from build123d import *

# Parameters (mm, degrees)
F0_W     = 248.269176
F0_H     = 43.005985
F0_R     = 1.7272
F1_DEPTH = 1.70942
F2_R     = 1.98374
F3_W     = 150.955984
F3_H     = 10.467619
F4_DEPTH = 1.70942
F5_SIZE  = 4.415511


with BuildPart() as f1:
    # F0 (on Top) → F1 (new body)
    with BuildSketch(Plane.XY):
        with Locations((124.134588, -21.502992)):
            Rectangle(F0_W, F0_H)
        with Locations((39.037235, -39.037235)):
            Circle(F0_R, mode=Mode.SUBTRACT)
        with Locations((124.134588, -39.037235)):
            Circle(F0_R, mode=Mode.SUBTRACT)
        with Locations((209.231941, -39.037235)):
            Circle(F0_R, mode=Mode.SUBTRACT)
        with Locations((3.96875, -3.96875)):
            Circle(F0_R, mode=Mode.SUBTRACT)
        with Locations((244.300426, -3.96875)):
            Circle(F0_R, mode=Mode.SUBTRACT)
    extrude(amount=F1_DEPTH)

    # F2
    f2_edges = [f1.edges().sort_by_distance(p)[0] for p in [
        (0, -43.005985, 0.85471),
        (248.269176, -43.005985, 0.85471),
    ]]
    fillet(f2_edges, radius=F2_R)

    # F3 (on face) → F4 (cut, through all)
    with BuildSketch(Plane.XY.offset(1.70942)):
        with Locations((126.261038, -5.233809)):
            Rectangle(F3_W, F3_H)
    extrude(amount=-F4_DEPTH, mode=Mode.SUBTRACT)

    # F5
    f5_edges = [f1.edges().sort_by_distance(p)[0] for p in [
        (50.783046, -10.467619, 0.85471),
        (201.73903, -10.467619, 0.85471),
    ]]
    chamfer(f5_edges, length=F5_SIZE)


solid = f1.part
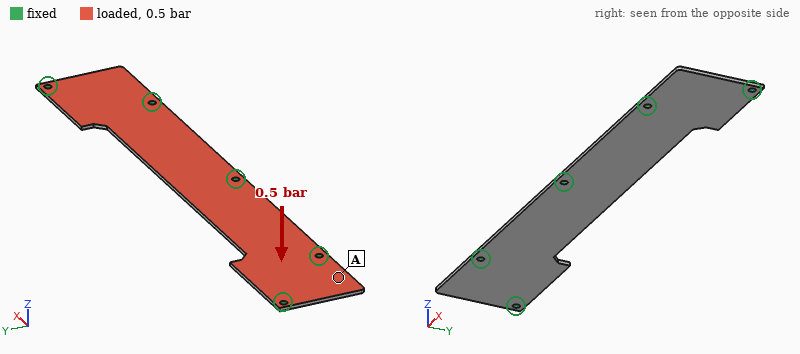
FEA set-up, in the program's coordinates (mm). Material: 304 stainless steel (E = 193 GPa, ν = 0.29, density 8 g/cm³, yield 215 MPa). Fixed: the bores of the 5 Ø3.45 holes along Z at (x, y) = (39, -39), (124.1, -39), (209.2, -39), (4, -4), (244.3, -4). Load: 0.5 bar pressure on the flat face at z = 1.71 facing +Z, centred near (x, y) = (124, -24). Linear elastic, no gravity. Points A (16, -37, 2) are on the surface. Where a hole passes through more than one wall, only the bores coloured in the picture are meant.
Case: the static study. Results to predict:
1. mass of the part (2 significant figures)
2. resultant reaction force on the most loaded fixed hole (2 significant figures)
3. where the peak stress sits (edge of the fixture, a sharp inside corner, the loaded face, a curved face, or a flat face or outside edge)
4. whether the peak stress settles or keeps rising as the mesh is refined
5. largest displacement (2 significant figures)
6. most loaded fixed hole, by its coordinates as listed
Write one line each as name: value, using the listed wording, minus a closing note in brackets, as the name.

mass of the part: 120 g
resultant reaction force on the most loaded fixed hole: 140 N
where the peak stress sits: edge of the fixture
whether the peak stress settles or keeps rising as the mesh is refined: keeps rising
largest displacement: 0.21 mm
most loaded fixed hole, by its coordinates as listed: (124.1, -39)
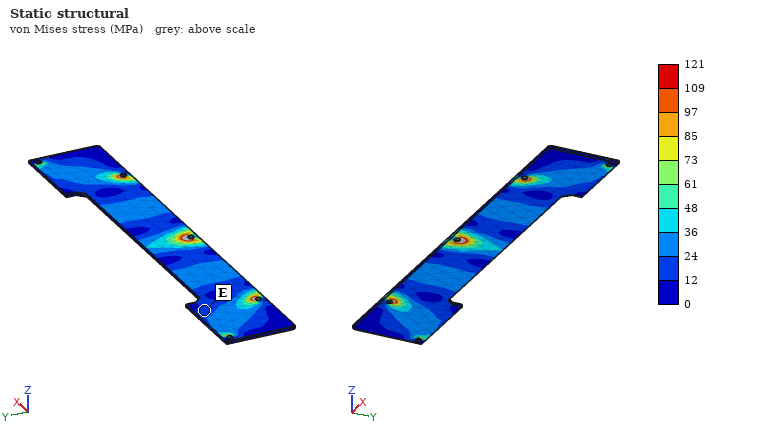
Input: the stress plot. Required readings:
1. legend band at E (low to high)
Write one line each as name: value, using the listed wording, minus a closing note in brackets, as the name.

legend band at E: 12 to 24 MPa
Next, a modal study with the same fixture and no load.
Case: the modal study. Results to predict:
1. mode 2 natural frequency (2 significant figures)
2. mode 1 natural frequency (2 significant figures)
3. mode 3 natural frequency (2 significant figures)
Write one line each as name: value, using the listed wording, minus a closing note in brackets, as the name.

mode 2 natural frequency: 880 Hz
mode 1 natural frequency: 870 Hz
mode 3 natural frequency: 1500 Hz
